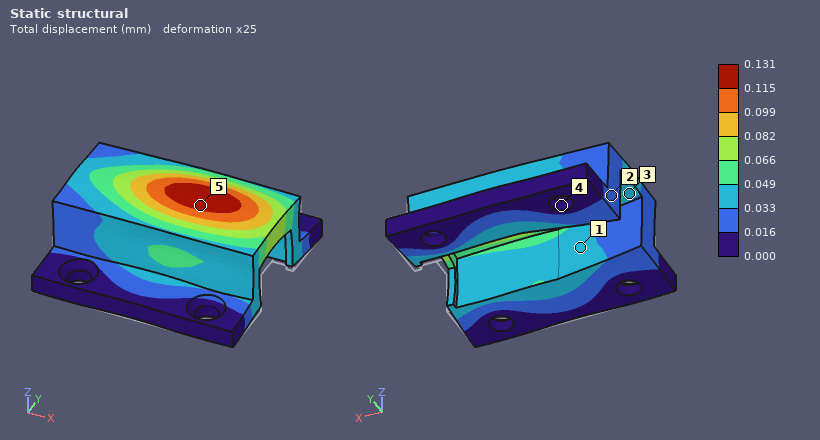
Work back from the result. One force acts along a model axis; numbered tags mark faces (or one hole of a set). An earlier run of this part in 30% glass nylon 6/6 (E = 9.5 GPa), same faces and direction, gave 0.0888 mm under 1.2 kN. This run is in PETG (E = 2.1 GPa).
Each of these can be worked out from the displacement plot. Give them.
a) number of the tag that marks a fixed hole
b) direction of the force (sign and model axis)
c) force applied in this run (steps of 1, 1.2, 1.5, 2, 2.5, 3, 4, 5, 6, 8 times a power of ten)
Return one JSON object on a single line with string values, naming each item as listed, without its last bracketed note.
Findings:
{"number of the tag that marks a fixed hole": "4", "direction of the force": "+Z", "force applied in this run": "400 N"}
